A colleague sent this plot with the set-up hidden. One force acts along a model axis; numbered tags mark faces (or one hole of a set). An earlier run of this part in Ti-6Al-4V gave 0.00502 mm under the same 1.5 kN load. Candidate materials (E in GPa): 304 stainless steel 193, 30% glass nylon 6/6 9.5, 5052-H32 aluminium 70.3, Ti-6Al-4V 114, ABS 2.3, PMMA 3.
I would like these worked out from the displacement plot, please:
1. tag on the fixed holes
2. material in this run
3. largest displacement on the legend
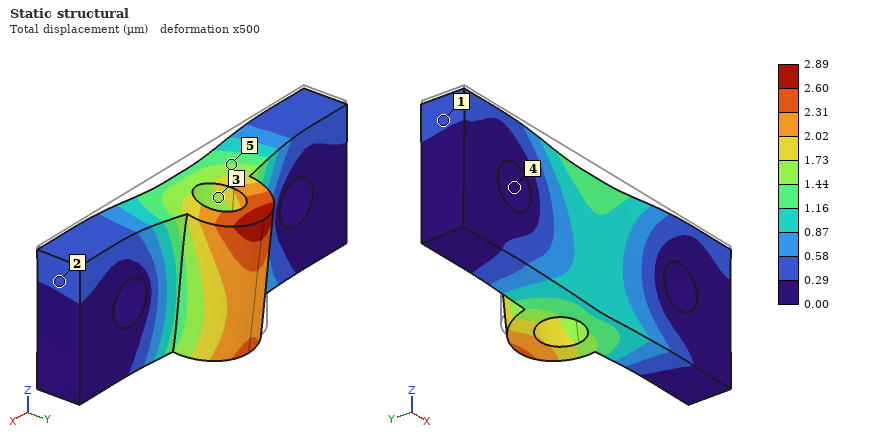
4
304 stainless steel
2.89 µm
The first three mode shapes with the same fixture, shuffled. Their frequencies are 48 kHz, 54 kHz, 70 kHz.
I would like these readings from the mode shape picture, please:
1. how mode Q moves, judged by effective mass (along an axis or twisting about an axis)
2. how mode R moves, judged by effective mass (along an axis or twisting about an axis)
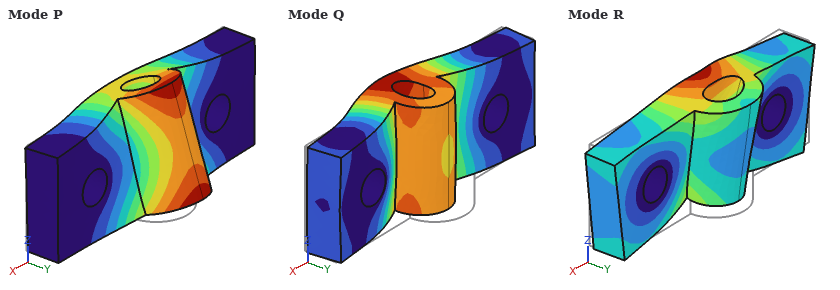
along Y
along Z
